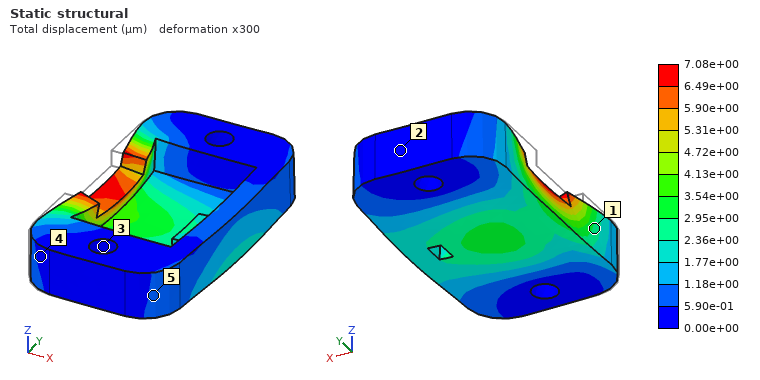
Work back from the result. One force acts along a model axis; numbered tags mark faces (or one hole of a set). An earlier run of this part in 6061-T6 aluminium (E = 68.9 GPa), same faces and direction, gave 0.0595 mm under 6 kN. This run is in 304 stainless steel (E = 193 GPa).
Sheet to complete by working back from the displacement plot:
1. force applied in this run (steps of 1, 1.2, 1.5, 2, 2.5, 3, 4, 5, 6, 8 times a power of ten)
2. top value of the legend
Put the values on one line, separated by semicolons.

2 kN; 7.08e+00 µm
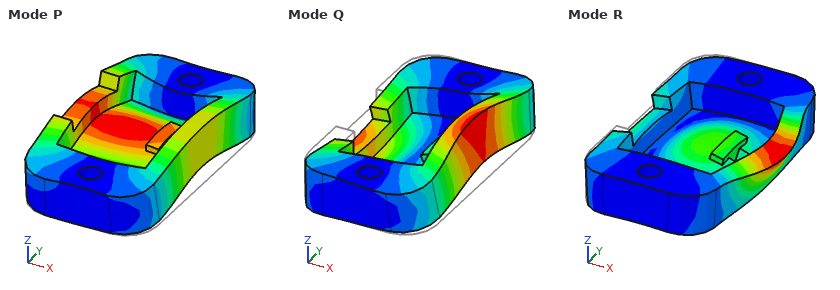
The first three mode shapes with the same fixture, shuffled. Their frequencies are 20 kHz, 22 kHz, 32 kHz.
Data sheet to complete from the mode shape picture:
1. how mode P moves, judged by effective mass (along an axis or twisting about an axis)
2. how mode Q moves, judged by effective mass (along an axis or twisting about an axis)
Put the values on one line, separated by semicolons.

along Z; twisting about Y
